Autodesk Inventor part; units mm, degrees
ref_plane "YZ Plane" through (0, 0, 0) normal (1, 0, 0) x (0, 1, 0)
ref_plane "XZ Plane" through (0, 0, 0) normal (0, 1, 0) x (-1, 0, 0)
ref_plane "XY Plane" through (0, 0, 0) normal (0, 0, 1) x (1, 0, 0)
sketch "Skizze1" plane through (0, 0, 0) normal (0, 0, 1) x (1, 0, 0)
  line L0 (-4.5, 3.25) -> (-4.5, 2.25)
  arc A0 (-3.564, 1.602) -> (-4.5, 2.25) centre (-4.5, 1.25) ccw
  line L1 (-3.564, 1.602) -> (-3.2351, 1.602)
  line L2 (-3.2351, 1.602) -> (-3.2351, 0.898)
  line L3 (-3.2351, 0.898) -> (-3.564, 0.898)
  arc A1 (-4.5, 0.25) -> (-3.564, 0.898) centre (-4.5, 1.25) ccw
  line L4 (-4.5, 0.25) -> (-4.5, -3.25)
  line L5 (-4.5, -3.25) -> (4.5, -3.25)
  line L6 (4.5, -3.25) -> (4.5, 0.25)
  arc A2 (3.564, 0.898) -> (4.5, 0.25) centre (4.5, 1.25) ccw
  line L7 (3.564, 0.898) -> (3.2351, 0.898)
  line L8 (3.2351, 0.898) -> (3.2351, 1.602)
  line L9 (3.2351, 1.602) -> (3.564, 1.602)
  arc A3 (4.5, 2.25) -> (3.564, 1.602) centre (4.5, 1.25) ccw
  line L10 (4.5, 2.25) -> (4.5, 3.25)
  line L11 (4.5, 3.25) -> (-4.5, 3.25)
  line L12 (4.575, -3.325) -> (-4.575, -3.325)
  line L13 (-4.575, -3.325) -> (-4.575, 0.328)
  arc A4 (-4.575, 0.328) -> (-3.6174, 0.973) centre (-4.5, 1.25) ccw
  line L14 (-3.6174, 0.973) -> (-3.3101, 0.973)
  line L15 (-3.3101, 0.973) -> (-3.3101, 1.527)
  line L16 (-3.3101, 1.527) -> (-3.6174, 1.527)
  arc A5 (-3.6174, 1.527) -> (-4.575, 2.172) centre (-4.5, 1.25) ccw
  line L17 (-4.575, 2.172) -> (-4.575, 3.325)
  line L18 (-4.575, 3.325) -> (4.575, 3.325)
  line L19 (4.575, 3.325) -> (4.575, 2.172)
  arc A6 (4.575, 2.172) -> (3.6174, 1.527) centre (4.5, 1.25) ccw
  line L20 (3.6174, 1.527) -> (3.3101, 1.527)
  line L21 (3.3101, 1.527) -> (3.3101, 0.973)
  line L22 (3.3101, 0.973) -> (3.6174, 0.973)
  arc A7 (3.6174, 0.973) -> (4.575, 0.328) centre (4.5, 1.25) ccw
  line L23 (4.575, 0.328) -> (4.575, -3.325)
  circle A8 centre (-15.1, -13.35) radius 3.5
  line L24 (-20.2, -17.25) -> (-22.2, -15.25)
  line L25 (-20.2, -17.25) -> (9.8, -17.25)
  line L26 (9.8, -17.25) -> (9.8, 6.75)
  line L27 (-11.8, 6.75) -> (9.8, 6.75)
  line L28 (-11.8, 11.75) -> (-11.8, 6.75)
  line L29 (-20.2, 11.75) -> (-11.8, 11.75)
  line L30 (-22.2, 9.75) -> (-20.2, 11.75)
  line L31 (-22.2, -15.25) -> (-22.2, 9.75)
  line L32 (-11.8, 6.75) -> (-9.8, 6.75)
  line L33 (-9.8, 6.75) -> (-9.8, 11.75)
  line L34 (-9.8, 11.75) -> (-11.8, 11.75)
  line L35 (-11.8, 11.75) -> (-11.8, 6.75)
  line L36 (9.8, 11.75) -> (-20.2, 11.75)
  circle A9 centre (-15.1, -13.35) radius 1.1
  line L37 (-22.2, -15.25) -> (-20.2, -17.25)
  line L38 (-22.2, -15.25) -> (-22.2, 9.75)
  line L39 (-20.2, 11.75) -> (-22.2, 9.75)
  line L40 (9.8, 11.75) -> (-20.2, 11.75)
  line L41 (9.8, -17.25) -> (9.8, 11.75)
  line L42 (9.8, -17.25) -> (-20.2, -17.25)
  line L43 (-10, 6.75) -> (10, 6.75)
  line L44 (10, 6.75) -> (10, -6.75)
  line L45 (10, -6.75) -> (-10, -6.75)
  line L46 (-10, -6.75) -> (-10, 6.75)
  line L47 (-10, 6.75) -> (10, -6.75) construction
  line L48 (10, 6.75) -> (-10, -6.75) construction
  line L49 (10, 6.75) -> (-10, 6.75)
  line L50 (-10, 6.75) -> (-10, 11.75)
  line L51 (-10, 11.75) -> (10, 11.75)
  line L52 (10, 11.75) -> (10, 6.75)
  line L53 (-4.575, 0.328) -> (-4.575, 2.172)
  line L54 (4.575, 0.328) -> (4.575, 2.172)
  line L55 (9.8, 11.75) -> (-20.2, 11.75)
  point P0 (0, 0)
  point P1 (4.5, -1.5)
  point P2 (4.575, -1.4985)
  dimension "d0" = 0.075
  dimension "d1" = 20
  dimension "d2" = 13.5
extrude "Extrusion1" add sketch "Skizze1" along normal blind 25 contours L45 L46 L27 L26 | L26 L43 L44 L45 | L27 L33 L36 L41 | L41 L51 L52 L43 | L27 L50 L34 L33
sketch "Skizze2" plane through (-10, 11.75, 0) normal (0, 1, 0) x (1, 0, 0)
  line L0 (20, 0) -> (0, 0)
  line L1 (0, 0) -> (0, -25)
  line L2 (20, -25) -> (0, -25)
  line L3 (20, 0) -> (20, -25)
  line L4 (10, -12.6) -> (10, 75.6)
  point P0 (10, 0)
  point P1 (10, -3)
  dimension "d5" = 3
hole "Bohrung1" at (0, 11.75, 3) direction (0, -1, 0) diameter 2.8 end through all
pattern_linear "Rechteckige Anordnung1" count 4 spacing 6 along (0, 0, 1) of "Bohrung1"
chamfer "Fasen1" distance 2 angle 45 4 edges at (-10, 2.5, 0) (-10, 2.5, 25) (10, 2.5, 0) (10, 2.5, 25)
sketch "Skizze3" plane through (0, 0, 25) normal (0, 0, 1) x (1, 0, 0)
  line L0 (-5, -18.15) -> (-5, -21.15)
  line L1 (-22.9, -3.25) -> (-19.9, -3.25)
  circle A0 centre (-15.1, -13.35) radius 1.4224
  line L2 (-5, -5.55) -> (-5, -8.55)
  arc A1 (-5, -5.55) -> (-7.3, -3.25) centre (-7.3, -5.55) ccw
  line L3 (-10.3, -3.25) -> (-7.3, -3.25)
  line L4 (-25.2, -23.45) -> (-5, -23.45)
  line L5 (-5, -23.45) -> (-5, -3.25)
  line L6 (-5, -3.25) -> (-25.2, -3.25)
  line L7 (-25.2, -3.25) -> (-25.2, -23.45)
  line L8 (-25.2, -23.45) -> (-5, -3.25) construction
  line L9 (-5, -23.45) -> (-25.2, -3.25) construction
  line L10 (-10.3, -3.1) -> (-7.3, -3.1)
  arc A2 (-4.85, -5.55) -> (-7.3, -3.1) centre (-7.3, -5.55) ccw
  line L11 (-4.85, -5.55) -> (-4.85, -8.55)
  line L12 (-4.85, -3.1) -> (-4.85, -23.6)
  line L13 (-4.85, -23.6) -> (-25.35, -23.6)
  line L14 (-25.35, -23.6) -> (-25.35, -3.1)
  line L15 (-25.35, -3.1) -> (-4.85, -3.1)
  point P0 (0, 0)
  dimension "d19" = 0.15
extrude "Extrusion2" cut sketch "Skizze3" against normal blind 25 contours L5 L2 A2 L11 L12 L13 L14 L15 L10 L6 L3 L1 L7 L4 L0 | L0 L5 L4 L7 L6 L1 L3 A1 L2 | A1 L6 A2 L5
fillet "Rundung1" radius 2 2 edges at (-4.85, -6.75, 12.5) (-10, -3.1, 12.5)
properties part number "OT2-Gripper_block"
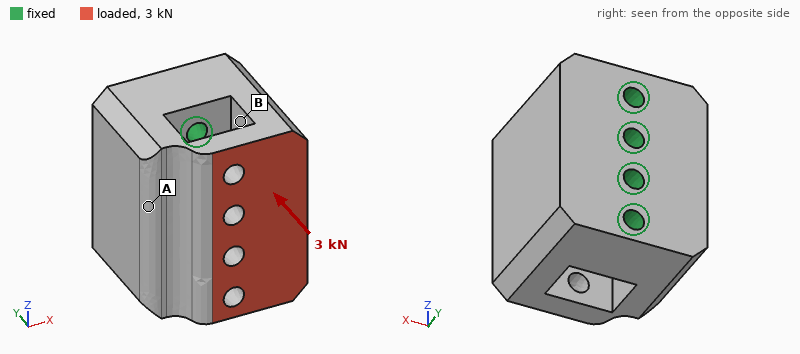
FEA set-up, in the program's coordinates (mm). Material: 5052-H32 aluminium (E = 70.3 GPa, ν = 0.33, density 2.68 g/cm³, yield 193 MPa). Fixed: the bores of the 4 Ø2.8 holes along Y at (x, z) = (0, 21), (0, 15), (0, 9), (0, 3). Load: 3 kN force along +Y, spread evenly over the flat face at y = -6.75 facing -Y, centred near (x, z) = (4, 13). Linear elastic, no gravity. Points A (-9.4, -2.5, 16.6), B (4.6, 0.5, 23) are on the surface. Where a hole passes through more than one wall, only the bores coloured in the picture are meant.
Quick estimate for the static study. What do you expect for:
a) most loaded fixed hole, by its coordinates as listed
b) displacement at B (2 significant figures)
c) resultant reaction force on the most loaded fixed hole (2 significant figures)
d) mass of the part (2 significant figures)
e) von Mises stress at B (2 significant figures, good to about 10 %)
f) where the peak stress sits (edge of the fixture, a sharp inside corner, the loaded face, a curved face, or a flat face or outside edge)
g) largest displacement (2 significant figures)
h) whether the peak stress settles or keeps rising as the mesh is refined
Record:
(0, 21)
6.5 µm
840 N
18 g
39 MPa
edge of the fixture
12 µm
keeps rising
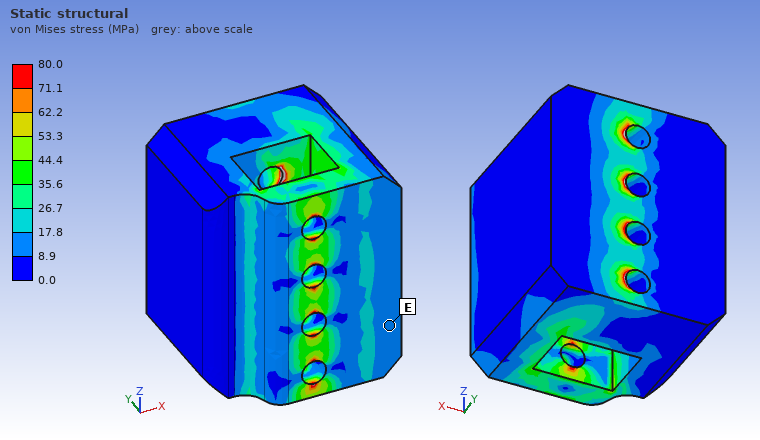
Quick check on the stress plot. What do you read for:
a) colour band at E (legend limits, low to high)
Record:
8.9 to 17.8 MPa
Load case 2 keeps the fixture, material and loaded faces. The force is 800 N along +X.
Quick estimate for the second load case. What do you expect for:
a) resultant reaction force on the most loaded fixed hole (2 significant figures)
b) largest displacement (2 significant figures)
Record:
240 N
12 µm
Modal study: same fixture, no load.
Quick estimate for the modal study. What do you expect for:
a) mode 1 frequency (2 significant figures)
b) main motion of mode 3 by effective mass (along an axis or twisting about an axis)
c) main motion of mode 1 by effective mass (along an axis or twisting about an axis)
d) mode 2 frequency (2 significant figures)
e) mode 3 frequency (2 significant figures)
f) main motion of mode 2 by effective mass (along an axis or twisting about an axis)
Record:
21 kHz
twisting about Y
along X
29 kHz
38 kHz
along Z
